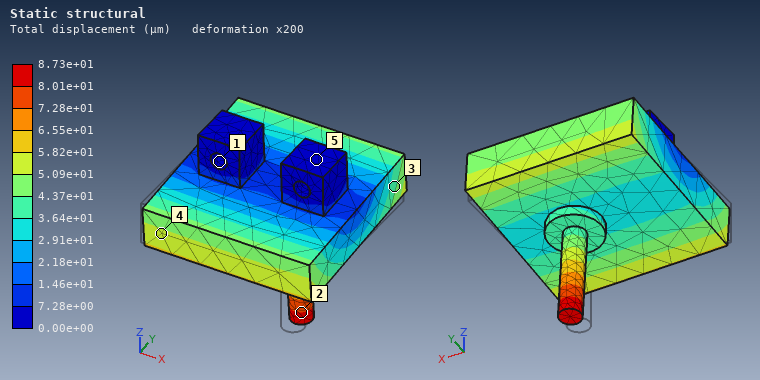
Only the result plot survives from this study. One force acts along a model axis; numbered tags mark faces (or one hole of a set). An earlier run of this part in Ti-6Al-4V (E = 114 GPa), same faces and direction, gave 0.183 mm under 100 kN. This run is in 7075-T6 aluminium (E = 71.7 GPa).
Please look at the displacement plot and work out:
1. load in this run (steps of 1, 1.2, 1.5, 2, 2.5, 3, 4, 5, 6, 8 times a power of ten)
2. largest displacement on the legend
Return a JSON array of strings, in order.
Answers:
["30 kN", "8.73e+01 µm"]
